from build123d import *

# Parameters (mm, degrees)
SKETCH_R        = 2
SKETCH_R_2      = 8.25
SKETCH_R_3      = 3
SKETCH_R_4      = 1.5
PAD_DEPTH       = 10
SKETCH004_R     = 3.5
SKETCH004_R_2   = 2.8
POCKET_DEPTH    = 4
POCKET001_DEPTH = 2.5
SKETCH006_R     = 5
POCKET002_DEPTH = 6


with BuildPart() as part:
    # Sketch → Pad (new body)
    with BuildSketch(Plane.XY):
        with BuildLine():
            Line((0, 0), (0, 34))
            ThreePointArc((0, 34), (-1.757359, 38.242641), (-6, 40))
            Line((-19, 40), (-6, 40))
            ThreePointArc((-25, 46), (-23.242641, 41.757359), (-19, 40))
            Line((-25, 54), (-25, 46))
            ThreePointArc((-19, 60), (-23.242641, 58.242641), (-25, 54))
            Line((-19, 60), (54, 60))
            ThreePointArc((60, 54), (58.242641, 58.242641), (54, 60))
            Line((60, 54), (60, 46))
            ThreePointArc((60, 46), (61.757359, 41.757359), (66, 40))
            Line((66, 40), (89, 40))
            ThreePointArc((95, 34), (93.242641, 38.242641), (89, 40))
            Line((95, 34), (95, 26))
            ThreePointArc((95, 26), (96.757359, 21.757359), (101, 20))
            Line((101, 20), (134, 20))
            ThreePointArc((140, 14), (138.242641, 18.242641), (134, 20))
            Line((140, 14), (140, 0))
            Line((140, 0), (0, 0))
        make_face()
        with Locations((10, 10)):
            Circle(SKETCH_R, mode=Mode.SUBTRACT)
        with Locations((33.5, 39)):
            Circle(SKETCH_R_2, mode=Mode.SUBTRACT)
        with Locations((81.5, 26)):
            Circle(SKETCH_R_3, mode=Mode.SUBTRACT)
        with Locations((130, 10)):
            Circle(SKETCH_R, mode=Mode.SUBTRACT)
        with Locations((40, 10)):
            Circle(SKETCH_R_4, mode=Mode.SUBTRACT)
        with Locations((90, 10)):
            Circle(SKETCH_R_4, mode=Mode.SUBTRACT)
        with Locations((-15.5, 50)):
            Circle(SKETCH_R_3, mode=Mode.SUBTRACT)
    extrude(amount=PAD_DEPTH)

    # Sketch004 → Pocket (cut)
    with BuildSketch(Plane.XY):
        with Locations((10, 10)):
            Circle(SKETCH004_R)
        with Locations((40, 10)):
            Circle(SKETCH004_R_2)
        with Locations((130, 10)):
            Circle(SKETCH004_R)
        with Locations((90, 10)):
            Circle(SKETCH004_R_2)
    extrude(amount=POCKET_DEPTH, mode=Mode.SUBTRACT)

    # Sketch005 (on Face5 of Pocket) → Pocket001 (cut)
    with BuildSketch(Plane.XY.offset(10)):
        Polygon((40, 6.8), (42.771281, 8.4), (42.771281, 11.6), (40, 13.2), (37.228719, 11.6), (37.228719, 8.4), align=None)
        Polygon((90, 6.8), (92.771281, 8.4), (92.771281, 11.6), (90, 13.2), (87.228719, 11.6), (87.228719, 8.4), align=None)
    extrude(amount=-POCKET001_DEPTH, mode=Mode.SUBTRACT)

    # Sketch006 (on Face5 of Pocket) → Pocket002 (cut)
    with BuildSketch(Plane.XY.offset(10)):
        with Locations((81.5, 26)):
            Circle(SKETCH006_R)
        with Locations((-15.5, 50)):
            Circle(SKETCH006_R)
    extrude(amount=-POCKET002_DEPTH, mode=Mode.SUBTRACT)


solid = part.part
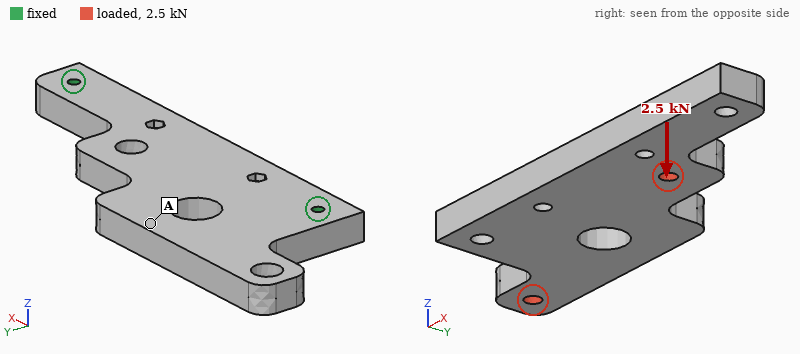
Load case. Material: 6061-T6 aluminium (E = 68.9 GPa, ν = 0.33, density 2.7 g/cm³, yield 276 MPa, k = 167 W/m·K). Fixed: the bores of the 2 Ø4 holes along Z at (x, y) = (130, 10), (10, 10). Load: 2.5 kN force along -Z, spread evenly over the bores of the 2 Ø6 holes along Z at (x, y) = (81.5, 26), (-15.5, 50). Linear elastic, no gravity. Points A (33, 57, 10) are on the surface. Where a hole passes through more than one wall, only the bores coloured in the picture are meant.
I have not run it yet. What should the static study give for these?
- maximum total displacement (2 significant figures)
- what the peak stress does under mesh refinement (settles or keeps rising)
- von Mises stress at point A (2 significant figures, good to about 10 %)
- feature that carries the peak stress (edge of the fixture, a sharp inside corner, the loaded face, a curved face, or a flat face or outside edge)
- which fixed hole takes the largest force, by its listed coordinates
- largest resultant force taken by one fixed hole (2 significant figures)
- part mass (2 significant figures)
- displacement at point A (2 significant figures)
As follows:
0.65 mm
keeps rising
38 MPa
edge of the fixture
(10, 10)
2.0 kN
160 g
0.39 mm
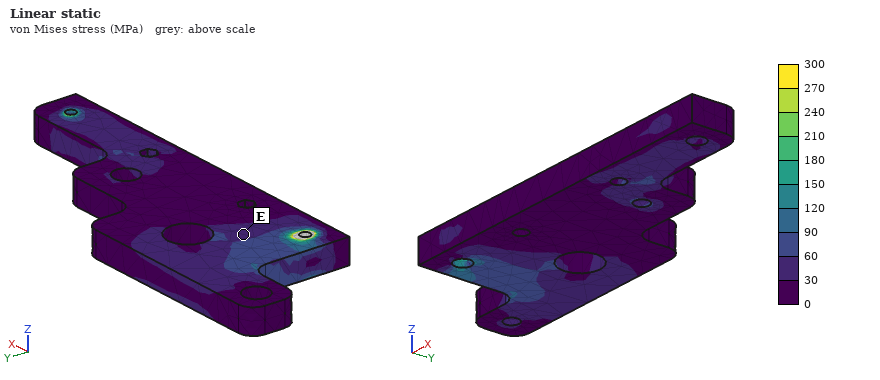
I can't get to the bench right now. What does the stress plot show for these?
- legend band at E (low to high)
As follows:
30 to 60 MPa
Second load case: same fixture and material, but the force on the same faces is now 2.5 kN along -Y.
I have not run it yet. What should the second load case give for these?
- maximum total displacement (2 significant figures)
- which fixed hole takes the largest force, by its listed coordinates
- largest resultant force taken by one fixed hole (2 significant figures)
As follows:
88 µm
(10, 10)
2.0 kN
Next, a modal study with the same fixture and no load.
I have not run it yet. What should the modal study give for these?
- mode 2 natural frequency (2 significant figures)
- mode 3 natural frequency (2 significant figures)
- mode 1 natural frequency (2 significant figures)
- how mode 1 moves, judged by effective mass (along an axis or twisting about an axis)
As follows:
2200 Hz
3800 Hz
1400 Hz
along Z
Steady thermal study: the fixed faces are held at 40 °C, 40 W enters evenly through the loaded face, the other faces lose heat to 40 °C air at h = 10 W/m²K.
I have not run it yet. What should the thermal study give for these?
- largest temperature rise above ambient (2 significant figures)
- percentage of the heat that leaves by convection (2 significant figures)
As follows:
38 K
6.4 %
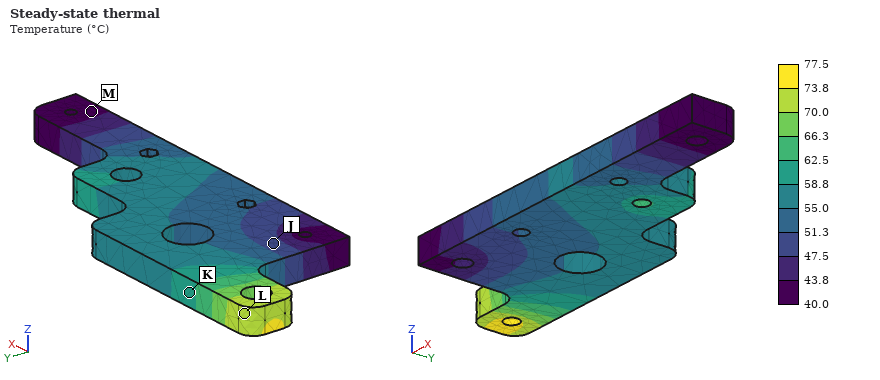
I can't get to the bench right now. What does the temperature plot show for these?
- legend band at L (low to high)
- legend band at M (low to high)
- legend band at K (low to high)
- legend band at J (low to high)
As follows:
70.0 to 73.8 °C
40.0 to 43.8 °C
58.8 to 62.5 °C
47.5 to 51.3 °C
